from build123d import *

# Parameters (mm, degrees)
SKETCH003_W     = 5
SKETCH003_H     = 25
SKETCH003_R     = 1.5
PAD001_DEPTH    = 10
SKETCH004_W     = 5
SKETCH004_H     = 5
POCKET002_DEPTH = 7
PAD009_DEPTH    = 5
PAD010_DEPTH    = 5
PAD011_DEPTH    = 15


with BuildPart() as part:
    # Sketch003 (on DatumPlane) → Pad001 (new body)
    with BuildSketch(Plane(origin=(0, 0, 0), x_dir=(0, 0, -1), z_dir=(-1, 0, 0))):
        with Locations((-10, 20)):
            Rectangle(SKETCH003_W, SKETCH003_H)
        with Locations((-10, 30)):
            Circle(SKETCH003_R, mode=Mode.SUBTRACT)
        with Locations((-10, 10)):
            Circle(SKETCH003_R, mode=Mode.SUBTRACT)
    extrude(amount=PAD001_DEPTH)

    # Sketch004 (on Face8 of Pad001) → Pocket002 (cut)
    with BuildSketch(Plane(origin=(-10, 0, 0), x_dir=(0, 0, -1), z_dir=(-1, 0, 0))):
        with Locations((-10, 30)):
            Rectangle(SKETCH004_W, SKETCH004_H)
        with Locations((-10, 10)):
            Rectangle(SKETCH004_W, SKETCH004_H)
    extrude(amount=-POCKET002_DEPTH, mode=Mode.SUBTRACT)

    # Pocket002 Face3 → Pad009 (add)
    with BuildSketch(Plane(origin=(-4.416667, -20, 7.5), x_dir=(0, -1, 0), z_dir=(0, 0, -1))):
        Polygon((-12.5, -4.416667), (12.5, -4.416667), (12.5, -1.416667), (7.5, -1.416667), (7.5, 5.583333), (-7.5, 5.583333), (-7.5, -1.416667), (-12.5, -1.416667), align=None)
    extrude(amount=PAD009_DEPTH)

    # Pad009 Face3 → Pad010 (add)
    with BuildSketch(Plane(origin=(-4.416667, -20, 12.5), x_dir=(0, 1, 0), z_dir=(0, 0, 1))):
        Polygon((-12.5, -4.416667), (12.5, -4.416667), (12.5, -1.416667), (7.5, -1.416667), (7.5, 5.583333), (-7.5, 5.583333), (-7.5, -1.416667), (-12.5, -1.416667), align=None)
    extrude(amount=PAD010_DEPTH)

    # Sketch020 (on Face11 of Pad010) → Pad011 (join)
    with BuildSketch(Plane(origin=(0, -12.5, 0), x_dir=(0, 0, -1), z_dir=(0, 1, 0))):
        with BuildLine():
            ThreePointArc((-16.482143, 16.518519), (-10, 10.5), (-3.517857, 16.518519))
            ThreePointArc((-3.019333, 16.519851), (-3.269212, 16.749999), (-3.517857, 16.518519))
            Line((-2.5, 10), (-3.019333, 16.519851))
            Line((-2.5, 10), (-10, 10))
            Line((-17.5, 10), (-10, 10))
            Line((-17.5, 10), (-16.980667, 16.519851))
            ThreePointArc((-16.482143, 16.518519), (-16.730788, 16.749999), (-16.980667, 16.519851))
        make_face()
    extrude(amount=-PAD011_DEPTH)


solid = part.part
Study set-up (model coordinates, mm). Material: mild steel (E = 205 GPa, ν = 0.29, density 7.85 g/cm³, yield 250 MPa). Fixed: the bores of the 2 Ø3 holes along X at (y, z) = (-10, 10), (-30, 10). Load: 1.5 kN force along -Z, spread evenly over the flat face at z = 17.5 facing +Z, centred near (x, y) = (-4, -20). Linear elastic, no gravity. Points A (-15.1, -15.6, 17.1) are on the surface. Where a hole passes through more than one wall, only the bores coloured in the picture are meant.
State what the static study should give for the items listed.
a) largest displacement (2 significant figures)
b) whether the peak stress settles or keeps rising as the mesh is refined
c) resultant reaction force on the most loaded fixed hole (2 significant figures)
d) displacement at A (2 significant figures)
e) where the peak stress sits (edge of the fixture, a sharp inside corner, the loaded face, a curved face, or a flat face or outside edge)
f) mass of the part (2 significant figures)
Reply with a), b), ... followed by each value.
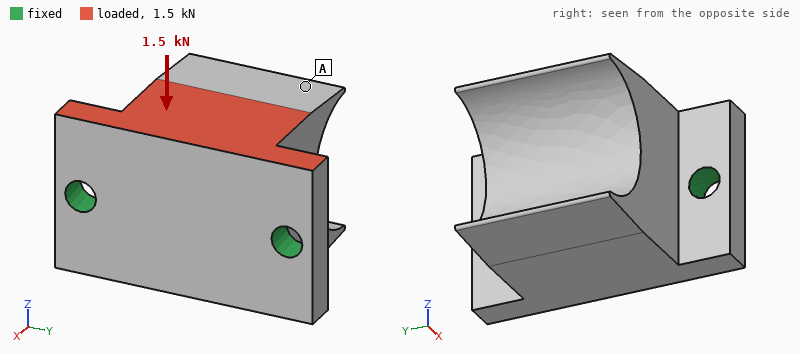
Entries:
a) 14 µm
b) keeps rising
c) 750 N
d) 13 µm
e) edge of the fixture
f) 25 g
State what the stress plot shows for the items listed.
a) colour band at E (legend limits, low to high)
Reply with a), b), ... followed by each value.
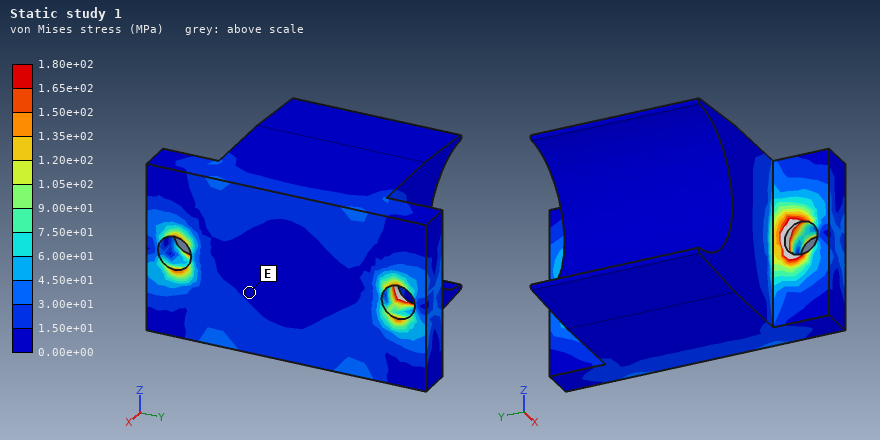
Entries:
a) 0.00e+00 to 1.50e+01 MPa
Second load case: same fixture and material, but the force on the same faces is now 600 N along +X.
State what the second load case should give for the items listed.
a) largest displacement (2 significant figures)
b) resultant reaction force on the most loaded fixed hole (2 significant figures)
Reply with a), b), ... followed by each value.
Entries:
a) 13 µm
b) 320 N
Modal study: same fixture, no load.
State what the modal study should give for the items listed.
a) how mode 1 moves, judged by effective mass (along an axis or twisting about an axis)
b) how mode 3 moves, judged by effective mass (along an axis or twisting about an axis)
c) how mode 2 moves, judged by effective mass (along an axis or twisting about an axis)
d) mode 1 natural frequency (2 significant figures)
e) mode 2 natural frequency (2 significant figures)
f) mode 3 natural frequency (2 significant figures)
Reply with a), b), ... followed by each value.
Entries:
a) along Z
b) along Y
c) along X
d) 11 kHz
e) 28 kHz
f) 30 kHz
